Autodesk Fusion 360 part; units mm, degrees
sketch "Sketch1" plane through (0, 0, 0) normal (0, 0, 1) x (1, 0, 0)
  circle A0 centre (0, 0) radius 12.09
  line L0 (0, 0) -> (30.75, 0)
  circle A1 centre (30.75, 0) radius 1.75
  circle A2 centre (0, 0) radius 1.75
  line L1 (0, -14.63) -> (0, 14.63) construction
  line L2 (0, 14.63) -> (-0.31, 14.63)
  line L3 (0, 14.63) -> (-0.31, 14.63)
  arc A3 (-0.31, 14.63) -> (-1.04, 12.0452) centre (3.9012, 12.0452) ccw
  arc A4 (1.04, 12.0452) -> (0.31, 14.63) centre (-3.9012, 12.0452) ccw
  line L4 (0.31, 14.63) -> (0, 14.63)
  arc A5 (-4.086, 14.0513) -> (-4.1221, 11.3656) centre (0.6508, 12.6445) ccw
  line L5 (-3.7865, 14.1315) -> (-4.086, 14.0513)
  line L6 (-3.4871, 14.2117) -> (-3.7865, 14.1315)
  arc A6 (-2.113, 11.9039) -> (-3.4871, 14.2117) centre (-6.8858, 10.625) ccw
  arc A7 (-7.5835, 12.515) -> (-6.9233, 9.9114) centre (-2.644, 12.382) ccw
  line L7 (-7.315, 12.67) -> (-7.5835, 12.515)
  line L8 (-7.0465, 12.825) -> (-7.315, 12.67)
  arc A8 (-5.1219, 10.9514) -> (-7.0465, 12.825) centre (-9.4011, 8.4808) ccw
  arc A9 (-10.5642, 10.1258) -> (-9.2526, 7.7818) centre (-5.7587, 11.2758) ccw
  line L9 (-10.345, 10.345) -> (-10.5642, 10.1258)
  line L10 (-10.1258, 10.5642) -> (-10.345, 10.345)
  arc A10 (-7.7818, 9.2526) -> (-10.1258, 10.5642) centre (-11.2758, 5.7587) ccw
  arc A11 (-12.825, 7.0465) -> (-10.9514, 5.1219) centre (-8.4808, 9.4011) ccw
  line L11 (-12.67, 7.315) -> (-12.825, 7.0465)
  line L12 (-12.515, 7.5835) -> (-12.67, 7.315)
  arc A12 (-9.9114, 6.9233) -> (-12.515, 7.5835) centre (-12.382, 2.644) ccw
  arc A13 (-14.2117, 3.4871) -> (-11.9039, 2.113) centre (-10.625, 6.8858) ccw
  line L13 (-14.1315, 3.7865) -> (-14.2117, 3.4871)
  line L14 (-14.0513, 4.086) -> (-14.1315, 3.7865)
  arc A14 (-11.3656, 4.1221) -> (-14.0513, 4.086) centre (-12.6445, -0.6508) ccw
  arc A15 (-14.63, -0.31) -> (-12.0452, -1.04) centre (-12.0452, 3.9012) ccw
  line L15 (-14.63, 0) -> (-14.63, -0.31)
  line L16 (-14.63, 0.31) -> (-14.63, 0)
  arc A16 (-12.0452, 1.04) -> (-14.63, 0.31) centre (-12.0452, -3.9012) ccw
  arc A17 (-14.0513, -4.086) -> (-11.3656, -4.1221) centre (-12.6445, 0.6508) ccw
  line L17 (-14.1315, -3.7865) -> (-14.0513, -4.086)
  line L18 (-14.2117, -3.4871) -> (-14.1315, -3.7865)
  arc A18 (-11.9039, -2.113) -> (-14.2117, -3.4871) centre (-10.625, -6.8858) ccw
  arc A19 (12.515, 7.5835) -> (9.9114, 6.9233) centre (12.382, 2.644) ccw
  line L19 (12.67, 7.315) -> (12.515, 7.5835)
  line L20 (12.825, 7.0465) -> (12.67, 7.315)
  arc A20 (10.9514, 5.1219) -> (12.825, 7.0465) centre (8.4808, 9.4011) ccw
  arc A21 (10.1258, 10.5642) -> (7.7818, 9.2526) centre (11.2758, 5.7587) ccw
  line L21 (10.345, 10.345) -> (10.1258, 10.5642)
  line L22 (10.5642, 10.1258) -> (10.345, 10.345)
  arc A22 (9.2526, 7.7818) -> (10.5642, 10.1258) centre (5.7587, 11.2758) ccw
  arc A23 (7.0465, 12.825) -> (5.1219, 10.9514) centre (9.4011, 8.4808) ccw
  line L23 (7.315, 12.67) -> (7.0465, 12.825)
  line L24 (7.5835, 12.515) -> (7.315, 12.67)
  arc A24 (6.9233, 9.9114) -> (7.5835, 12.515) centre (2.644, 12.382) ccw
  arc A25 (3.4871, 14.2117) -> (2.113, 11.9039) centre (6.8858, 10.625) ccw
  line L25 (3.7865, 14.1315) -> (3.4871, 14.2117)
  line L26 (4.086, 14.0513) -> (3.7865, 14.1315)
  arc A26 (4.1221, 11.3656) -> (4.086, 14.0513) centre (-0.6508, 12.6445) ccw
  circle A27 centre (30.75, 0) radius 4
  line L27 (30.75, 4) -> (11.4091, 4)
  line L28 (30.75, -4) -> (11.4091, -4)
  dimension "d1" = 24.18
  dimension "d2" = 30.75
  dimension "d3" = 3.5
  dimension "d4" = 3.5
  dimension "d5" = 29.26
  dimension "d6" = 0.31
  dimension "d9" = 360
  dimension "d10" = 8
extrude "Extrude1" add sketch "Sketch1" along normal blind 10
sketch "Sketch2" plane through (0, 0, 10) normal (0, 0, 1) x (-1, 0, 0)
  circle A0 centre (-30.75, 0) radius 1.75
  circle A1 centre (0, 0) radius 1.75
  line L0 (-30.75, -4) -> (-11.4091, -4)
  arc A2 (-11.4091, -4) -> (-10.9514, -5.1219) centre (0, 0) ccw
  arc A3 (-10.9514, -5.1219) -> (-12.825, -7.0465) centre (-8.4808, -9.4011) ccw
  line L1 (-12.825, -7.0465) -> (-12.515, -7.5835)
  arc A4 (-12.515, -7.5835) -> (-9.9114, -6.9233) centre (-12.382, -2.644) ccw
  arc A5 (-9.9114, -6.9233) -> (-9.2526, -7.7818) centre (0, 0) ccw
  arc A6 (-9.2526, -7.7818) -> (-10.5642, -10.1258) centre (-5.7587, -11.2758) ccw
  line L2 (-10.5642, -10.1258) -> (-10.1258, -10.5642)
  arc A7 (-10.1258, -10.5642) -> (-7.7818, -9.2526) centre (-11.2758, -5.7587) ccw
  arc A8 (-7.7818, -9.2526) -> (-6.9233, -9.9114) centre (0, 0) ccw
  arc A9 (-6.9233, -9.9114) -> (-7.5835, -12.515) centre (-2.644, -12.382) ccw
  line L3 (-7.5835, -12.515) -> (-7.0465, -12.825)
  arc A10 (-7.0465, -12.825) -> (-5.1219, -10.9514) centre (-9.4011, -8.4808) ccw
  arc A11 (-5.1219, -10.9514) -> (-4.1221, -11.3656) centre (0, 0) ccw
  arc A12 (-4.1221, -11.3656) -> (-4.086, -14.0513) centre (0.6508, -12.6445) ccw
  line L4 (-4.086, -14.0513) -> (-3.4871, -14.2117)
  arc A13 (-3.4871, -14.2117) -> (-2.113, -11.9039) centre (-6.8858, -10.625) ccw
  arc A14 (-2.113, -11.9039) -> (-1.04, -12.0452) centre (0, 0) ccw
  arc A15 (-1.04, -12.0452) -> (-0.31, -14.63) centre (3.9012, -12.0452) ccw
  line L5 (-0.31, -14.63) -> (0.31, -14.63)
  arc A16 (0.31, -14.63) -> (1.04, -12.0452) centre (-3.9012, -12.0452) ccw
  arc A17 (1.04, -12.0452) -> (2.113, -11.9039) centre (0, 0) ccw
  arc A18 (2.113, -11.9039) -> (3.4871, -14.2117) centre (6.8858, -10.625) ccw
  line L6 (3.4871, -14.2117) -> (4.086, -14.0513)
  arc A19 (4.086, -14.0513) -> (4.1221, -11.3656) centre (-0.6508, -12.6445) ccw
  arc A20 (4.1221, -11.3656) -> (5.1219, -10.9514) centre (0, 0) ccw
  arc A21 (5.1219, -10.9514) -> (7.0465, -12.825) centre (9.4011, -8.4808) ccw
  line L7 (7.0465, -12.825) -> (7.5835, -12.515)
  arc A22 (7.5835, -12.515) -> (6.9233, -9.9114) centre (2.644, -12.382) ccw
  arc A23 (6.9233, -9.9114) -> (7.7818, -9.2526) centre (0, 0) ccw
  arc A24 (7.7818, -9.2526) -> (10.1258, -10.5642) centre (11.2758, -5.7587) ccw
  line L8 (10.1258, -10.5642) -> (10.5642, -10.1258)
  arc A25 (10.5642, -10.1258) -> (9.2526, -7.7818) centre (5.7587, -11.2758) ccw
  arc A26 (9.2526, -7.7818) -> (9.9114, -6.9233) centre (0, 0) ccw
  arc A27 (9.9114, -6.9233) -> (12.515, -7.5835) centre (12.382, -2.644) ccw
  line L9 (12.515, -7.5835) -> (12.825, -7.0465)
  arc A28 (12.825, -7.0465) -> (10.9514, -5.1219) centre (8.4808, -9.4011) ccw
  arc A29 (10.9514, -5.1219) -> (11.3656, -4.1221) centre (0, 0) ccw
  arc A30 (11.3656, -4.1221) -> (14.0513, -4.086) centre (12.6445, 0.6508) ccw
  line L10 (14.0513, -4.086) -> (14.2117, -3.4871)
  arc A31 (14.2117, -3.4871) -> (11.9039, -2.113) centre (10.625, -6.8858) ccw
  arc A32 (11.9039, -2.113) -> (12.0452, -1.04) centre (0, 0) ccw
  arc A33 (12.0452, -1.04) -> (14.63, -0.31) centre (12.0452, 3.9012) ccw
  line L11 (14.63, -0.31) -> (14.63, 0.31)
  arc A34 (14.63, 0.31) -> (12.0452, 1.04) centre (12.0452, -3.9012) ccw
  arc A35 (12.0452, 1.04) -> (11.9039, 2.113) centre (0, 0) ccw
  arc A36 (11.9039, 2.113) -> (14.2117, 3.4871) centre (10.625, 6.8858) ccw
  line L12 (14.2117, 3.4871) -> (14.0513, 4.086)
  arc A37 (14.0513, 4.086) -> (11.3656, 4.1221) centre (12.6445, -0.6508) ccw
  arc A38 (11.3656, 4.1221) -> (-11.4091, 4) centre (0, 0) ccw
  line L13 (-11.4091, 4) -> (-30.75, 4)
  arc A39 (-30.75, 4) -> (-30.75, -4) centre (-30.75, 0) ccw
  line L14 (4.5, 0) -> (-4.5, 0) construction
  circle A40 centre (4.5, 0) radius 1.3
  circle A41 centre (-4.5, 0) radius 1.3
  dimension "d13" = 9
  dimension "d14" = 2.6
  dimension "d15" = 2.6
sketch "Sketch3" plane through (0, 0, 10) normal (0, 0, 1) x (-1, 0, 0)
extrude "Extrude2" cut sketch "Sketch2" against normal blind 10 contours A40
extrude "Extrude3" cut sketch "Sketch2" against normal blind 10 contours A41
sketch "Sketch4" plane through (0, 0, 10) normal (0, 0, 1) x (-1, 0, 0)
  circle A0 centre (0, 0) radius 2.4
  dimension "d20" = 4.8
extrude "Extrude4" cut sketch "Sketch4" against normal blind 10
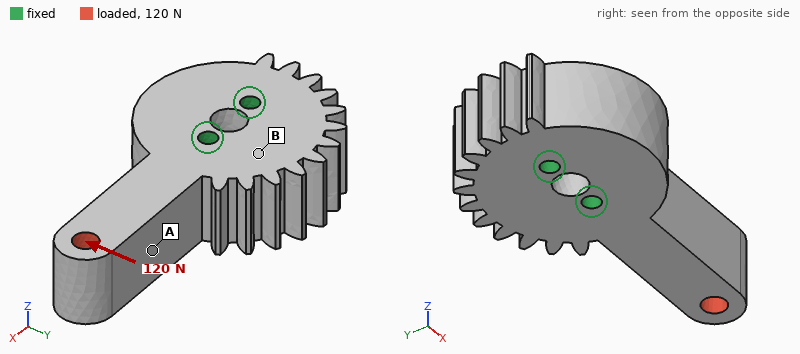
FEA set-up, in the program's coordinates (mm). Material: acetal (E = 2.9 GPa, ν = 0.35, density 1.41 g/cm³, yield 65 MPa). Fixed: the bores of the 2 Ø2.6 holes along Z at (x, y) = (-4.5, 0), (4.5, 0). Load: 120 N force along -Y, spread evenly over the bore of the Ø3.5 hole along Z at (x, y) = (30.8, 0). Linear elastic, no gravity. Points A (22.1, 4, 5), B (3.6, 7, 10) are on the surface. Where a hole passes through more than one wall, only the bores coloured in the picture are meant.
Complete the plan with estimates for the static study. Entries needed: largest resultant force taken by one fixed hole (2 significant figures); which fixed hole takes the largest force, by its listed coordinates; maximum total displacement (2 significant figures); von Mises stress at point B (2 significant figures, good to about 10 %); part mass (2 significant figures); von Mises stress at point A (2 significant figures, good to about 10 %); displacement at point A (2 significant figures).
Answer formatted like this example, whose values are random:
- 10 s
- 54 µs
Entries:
- 350 N
- (4.5, 0)
- 0.55 mm
- 3.6 MPa
- 9.1 g
- 9.8 MPa
- 0.24 mm
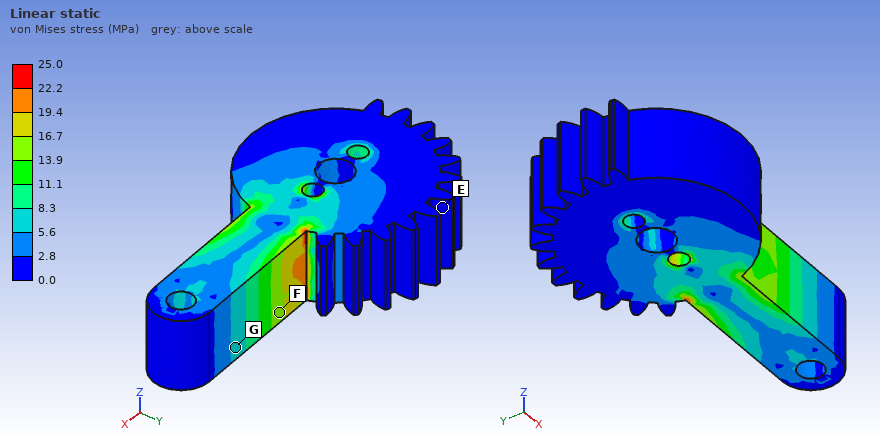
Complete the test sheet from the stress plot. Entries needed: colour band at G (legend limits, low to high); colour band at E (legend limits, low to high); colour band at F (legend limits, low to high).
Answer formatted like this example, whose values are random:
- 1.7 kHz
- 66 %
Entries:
- 5.6 to 8.3 MPa
- 0.0 to 2.8 MPa
- 13.9 to 16.7 MPa
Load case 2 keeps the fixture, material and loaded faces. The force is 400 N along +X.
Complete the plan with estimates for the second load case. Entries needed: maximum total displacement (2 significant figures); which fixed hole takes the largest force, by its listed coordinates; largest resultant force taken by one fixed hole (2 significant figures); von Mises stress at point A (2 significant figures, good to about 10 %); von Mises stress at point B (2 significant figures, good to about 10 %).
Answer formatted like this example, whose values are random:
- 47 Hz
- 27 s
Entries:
- 55 µm
- (4.5, 0)
- 330 N
- 5.2 MPa
- 0.96 MPa
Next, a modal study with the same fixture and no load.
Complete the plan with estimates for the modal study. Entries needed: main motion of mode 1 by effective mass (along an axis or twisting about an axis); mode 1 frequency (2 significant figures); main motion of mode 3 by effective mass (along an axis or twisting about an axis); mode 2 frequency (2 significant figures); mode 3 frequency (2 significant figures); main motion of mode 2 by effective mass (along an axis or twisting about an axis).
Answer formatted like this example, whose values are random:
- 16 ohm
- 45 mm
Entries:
- along Y
- 2600 Hz
- twisting about X
- 2800 Hz
- 7800 Hz
- along Z
